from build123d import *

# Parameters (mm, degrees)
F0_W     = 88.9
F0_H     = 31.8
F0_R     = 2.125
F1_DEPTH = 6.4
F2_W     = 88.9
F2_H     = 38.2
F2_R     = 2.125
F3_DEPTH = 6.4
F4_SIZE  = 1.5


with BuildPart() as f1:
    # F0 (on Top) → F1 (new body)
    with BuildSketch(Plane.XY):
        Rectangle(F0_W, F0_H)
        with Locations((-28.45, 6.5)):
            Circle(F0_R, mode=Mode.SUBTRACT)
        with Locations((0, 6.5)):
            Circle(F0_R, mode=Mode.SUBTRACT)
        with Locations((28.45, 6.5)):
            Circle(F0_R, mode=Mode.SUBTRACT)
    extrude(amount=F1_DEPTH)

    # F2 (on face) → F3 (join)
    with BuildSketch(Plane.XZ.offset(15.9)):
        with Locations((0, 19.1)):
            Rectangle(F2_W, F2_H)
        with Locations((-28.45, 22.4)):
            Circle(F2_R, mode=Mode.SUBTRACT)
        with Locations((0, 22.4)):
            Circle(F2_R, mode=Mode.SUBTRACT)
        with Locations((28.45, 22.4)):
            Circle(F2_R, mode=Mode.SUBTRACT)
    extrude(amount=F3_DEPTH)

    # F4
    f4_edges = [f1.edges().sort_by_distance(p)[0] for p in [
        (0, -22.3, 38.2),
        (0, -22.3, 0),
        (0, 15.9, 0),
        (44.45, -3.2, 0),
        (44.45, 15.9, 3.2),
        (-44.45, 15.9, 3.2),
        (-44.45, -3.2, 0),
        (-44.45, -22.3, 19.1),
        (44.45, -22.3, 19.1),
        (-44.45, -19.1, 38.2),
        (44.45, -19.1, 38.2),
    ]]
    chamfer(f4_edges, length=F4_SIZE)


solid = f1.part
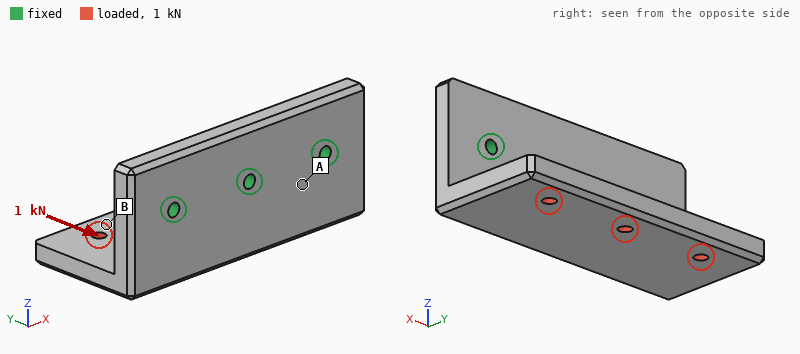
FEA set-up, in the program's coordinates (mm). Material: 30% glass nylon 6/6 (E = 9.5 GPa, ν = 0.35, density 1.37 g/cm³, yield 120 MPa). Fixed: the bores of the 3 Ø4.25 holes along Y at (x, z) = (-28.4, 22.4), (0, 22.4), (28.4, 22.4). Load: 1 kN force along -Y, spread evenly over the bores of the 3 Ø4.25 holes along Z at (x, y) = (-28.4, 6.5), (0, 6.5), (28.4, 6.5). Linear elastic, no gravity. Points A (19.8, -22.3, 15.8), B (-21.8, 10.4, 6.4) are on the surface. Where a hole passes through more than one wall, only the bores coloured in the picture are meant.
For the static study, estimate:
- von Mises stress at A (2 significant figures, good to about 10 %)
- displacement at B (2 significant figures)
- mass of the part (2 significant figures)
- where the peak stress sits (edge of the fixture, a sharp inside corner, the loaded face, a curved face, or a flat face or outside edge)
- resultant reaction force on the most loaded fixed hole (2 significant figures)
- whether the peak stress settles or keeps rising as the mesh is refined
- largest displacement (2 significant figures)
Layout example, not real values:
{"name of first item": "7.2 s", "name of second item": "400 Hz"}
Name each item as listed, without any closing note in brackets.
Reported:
{"von Mises stress at A": "16 MPa", "displacement at B": "0.37 mm", "mass of the part": "53 g", "where the peak stress sits": "edge of the fixture", "resultant reaction force on the most loaded fixed hole": "340 N", "whether the peak stress settles or keeps rising as the mesh is refined": "keeps rising", "largest displacement": "0.46 mm"}
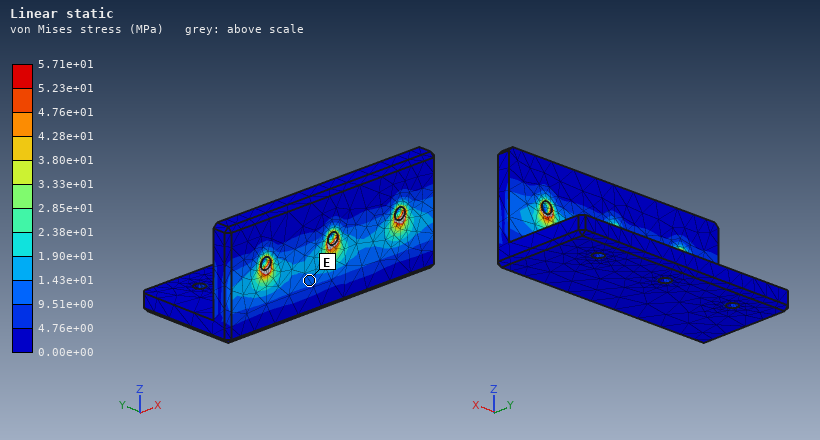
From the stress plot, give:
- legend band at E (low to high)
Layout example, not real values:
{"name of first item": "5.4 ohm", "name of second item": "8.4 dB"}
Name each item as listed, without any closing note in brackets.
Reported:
{"legend band at E": "9.51e+00 to 1.43e+01 MPa"}
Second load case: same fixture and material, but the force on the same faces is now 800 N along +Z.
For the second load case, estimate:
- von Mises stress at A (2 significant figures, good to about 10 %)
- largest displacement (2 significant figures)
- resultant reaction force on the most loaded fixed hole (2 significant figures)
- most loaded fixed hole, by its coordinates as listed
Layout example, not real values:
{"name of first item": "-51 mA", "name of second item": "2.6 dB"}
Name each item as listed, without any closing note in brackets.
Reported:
{"von Mises stress at A": "27 MPa", "largest displacement": "1.1 mm", "resultant reaction force on the most loaded fixed hole": "320 N", "most loaded fixed hole, by its coordinates as listed": "(0, 22.4)"}
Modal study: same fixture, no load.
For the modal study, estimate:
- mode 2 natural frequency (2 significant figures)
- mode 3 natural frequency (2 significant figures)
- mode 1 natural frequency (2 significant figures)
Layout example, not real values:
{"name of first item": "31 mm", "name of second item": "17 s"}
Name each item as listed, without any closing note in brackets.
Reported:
{"mode 2 natural frequency": "1800 Hz", "mode 3 natural frequency": "3100 Hz", "mode 1 natural frequency": "1200 Hz"}
